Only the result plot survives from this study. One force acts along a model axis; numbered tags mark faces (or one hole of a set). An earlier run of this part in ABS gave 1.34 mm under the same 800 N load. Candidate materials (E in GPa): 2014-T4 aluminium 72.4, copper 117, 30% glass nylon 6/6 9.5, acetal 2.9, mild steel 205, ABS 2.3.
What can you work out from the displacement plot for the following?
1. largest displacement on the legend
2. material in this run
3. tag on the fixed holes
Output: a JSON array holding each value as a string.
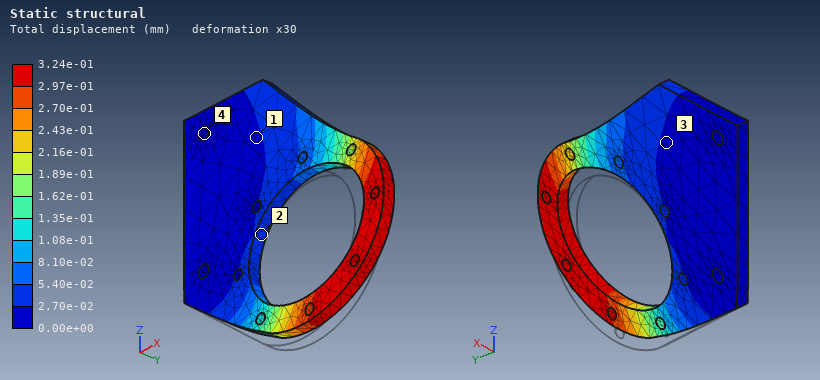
["3.24e-01 mm", "30% glass nylon 6/6", "4"]
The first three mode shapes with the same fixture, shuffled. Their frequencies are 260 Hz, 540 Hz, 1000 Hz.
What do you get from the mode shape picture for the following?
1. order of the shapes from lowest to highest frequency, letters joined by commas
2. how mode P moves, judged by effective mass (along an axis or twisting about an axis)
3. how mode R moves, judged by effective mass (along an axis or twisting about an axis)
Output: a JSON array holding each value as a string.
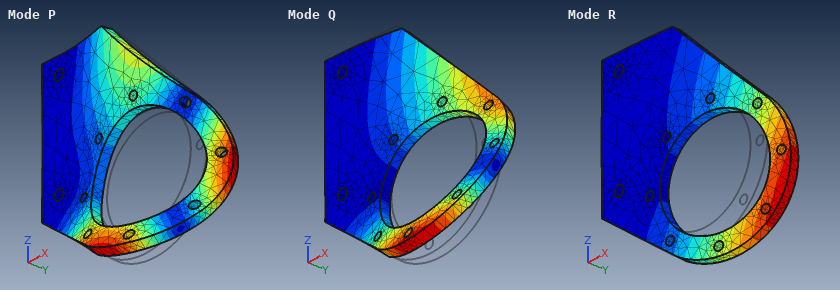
["R, Q, P", "along Y", "along Y"]
